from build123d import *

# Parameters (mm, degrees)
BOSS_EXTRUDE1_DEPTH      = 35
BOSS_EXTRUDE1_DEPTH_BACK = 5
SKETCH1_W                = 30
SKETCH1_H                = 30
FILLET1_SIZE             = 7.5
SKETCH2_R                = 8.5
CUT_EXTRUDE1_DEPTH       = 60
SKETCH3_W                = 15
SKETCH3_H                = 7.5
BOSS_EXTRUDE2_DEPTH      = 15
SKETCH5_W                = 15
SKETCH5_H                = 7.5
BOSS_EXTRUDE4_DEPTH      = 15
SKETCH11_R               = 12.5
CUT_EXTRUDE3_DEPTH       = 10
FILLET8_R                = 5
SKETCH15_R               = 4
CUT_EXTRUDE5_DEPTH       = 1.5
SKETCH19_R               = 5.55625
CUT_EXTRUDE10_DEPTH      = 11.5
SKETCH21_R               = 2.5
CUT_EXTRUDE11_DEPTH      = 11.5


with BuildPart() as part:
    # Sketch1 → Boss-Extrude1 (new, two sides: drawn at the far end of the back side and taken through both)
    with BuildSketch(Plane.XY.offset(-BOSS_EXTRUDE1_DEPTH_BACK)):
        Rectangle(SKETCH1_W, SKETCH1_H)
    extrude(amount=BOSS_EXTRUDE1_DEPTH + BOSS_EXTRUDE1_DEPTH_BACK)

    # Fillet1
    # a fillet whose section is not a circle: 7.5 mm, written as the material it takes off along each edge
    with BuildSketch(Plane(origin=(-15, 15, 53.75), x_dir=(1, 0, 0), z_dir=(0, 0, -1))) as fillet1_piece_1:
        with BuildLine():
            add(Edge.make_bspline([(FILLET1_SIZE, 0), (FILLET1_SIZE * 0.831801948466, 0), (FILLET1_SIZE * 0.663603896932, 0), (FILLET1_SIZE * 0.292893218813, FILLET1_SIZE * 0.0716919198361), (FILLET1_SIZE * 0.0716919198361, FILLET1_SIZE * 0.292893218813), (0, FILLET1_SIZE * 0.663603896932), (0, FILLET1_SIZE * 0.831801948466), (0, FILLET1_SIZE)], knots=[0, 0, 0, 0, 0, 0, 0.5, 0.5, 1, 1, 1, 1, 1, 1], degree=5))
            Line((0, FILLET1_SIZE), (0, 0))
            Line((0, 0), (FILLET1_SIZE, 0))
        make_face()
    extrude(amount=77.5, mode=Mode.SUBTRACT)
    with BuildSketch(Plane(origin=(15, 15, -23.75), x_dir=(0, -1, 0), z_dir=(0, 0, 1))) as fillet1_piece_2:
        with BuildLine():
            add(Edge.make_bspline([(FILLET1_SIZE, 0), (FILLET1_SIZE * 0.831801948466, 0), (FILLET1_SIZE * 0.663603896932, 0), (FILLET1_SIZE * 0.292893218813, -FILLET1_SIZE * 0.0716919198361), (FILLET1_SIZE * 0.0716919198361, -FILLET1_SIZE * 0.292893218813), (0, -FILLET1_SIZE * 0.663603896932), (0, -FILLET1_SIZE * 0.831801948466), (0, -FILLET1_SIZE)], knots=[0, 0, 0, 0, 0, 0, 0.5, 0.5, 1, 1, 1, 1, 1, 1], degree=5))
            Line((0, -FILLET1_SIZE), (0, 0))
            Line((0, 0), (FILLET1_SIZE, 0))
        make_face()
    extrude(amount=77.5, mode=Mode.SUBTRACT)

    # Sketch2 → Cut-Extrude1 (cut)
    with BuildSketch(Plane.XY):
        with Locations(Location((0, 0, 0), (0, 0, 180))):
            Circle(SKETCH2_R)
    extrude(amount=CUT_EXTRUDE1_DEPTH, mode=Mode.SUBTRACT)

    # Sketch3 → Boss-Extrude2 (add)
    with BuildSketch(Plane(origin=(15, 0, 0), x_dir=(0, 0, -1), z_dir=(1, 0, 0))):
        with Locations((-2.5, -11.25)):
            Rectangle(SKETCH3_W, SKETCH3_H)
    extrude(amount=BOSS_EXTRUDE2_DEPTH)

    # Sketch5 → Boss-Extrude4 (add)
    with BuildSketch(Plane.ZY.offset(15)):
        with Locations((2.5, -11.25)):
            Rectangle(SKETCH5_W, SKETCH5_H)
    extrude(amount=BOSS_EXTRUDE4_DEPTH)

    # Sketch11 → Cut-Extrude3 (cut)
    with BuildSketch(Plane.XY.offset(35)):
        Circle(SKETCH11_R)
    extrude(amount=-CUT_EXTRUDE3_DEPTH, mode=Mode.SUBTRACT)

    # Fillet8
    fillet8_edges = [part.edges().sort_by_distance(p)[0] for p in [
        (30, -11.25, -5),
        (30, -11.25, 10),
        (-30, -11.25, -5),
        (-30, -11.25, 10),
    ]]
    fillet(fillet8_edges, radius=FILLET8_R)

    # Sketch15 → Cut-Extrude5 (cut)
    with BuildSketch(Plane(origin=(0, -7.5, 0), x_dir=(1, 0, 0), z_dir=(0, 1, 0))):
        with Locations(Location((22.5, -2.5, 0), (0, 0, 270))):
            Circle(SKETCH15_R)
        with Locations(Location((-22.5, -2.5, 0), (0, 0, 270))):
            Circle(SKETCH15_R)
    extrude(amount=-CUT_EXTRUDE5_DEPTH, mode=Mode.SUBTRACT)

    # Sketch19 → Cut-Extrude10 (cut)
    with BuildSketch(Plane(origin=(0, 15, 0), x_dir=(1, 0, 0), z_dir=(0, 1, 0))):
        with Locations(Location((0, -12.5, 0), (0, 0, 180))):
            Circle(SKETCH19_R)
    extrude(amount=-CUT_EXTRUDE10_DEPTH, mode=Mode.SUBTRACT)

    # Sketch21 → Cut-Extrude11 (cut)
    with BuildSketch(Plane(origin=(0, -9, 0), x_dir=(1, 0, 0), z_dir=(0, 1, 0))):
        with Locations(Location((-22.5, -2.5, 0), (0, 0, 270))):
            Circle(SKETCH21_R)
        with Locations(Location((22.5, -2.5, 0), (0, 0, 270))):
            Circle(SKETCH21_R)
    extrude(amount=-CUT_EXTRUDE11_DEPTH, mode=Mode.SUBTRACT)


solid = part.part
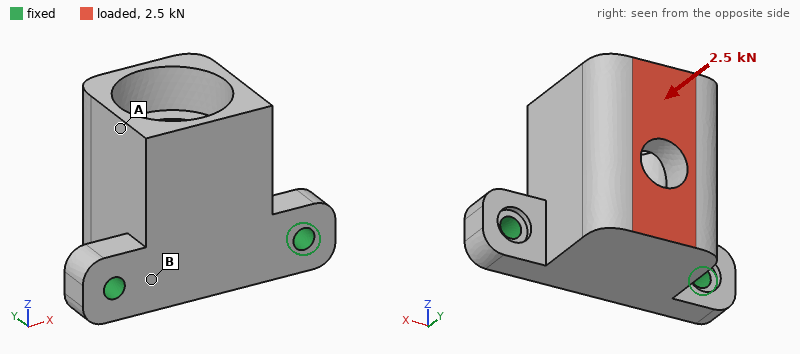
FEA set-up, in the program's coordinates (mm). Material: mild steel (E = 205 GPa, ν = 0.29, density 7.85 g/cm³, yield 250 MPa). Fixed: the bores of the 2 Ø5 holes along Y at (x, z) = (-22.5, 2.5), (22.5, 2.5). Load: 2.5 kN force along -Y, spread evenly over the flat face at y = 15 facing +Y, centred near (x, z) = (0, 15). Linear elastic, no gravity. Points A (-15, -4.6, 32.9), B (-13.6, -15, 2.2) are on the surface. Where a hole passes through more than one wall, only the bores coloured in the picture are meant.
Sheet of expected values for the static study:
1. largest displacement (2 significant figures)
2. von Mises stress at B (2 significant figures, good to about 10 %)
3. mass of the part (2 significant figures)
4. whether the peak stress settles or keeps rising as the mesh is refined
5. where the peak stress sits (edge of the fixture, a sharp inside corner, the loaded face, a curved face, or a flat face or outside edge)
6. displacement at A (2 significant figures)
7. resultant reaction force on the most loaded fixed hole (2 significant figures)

68 µm
63 MPa
210 g
keeps rising
edge of the fixture
48 µm
1.4 kN
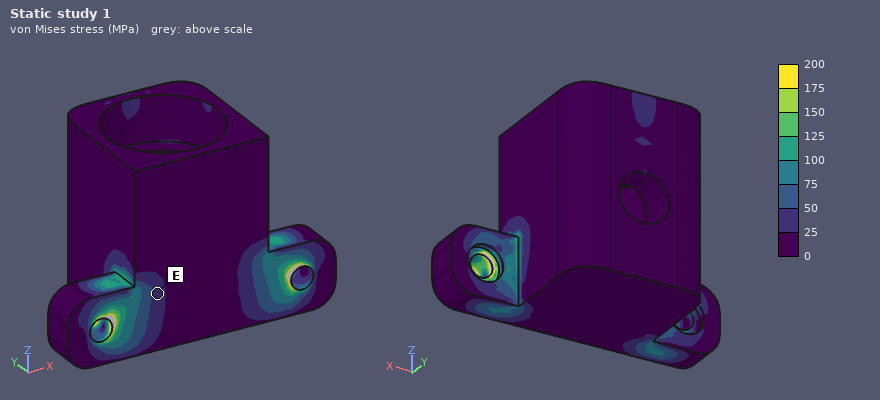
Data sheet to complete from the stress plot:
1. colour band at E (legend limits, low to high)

25 to 50 MPa
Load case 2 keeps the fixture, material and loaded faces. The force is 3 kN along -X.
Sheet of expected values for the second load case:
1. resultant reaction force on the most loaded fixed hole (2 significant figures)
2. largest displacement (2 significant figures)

2.8 kN
19 µm
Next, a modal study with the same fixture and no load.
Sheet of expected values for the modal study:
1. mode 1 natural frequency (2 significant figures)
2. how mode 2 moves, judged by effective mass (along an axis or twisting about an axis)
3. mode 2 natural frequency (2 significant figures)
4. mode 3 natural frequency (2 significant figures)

2600 Hz
along X
8600 Hz
10 kHz
